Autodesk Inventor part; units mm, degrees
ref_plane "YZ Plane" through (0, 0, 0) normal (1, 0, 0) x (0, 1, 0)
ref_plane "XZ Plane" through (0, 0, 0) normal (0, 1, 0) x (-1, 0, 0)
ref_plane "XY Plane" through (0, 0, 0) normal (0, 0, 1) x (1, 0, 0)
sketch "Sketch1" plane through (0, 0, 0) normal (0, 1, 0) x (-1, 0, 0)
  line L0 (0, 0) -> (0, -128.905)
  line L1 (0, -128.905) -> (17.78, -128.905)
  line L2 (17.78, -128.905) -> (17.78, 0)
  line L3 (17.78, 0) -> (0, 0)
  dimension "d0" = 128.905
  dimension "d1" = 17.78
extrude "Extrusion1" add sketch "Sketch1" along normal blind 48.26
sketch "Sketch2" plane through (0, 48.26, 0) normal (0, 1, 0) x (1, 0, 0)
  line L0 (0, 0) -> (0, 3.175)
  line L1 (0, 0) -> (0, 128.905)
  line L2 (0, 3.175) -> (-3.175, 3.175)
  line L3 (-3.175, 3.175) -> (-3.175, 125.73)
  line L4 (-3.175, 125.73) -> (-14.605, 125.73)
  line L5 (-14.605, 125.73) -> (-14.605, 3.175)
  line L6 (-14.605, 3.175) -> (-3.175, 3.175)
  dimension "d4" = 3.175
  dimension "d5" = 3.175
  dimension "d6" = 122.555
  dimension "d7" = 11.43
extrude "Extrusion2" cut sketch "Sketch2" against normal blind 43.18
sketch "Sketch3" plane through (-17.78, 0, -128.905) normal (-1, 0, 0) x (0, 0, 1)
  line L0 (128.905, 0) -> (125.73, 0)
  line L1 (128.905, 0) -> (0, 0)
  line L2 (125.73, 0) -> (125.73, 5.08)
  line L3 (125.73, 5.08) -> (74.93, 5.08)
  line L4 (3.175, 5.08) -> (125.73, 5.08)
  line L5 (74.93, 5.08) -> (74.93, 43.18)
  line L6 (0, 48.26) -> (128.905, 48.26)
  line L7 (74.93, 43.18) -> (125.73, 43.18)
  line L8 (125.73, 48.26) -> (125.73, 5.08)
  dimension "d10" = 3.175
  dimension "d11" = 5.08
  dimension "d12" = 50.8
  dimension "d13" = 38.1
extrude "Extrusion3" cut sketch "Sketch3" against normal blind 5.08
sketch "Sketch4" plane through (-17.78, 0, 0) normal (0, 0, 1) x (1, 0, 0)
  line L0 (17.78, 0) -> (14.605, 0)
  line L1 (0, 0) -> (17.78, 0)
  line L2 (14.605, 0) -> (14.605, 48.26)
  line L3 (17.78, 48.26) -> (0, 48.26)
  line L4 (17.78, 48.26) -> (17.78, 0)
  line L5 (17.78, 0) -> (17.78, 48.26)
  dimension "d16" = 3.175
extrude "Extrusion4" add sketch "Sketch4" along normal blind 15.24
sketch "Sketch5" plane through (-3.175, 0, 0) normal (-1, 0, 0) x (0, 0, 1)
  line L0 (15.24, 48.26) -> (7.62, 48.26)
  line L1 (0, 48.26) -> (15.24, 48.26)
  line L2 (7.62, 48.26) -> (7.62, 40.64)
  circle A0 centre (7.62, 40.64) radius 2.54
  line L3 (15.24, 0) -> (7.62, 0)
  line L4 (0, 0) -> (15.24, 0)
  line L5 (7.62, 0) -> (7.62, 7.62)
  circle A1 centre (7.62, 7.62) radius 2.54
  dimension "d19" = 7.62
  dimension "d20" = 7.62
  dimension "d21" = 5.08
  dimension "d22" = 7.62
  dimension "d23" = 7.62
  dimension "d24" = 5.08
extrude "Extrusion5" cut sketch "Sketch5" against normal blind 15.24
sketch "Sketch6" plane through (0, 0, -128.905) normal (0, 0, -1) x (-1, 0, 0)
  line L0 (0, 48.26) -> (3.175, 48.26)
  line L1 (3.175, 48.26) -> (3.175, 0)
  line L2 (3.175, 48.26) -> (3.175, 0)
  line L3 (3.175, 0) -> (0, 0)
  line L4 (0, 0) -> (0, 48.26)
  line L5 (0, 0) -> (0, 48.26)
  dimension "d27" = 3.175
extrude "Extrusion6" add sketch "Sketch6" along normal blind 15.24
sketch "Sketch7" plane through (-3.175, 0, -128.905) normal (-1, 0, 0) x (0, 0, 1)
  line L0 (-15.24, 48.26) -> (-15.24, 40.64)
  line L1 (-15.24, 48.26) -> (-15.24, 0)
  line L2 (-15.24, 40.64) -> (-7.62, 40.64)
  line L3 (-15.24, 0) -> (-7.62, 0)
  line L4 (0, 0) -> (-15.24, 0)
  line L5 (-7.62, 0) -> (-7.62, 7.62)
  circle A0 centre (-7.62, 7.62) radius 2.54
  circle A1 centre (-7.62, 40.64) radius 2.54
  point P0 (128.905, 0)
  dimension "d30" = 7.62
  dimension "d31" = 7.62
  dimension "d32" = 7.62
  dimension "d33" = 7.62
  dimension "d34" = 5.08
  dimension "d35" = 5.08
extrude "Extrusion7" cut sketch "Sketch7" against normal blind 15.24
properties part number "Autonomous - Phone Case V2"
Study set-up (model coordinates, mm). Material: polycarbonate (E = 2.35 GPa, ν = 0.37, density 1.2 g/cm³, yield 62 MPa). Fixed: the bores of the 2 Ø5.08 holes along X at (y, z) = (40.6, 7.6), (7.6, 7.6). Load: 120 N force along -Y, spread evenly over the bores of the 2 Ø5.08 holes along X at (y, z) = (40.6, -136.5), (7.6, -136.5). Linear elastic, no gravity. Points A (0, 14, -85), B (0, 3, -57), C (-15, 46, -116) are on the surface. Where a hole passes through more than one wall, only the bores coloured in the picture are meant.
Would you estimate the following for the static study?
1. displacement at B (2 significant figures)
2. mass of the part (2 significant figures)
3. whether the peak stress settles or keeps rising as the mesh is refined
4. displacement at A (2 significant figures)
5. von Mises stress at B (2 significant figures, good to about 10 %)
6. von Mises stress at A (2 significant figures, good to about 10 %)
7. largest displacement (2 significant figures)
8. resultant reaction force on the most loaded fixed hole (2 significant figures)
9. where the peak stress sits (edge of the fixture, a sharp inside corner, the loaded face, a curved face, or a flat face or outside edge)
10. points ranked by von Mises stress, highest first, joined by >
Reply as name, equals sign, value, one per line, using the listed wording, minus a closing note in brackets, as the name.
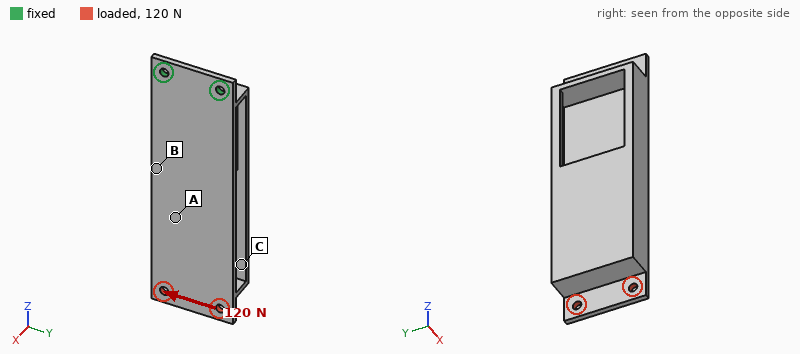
displacement at B = 0.55 mm
mass of the part = 58 g
whether the peak stress settles or keeps rising as the mesh is refined = keeps rising
displacement at A = 0.85 mm
von Mises stress at B = 4.7 MPa
von Mises stress at A = 2.4 MPa
largest displacement = 1.9 mm
resultant reaction force on the most loaded fixed hole = 500 N
where the peak stress sits = edge of the fixture
points ranked by von Mises stress, highest first, joined by > = B > A > C
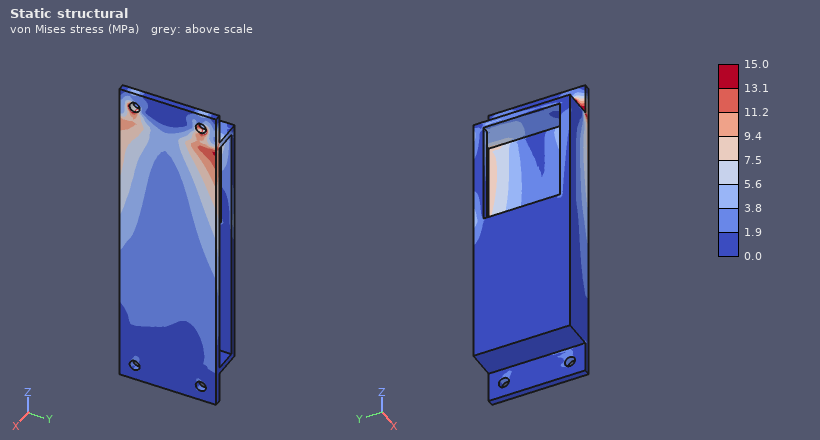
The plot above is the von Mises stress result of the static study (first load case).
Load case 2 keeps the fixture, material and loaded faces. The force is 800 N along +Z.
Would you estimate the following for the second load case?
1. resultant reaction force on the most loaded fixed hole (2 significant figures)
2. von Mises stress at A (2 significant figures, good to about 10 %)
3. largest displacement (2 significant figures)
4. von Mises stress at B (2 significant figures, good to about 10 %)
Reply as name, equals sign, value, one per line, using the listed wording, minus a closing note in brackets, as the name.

resultant reaction force on the most loaded fixed hole = 400 N
von Mises stress at A = 4.9 MPa
largest displacement = 1.7 mm
von Mises stress at B = 4.5 MPa
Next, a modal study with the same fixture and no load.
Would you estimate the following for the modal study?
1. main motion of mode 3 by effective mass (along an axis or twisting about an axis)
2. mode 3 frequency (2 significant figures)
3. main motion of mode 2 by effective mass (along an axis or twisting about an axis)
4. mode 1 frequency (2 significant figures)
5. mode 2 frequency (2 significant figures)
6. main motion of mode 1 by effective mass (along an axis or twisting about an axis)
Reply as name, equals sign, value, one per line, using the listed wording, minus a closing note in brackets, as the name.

main motion of mode 3 by effective mass = along Y
mode 3 frequency = 340 Hz
main motion of mode 2 by effective mass = along Y
mode 1 frequency = 40 Hz
mode 2 frequency = 200 Hz
main motion of mode 1 by effective mass = along X
